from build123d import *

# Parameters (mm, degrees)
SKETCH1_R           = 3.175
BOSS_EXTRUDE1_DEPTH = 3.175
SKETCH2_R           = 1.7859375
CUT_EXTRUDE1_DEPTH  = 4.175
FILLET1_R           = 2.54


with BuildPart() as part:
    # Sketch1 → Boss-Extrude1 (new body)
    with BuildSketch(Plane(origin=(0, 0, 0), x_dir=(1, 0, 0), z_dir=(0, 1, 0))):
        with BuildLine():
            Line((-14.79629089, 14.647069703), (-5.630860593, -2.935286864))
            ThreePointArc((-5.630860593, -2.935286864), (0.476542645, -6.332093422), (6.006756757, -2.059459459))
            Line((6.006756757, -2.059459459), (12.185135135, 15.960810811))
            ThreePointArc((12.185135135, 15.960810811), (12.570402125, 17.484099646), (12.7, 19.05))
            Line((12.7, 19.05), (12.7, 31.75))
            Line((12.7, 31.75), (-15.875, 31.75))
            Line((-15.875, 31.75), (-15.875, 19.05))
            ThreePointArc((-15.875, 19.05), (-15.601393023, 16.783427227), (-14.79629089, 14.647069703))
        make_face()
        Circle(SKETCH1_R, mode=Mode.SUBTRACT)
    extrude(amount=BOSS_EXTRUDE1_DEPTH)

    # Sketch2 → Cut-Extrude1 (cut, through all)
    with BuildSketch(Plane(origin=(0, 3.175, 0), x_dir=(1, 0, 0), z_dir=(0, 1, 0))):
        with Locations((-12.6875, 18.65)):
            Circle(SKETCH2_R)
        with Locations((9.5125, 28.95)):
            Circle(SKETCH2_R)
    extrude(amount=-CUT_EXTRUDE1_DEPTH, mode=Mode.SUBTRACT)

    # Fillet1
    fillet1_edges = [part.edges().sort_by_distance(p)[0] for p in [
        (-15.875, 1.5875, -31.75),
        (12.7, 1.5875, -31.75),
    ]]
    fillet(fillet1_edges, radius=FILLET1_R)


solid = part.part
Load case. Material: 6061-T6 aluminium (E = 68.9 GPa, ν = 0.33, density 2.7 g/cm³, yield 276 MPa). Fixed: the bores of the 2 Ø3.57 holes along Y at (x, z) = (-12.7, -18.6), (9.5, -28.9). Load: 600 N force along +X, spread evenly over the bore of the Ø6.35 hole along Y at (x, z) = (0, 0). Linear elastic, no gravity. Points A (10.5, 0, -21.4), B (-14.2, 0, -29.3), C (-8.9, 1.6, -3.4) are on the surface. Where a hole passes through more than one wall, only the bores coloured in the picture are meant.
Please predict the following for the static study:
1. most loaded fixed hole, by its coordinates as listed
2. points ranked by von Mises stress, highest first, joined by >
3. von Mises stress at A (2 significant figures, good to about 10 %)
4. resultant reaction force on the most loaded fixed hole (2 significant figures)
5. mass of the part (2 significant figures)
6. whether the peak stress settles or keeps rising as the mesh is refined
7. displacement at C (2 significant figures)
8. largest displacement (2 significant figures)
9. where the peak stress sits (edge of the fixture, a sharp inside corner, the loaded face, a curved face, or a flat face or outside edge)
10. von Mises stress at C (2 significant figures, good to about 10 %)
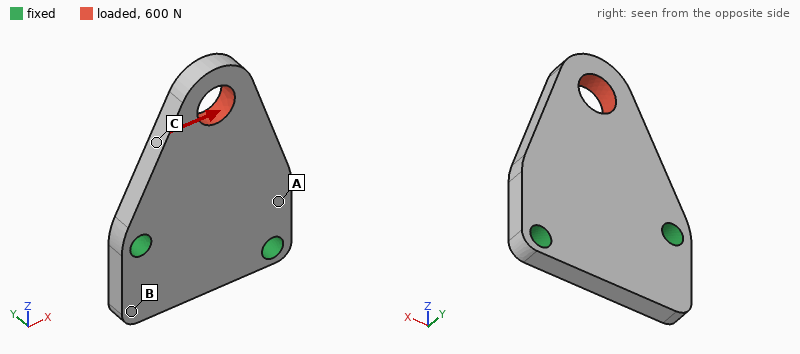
(-12.7, -18.6)
C > A > B
21 MPa
730 N
6.8 g
keeps rising
11 µm
22 µm
edge of the fixture
34 MPa
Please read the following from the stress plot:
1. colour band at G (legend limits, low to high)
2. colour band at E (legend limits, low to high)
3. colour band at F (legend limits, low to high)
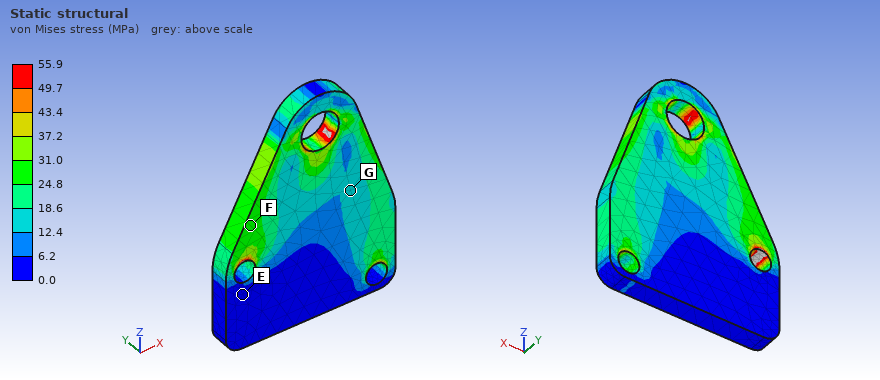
12.4 to 18.6 MPa
0.0 to 6.2 MPa
24.8 to 31.0 MPa
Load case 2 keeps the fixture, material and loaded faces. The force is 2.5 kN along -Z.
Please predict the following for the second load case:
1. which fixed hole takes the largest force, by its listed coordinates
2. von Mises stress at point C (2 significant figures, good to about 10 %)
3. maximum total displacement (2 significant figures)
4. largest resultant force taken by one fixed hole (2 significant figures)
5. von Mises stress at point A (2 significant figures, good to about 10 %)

(9.5, -28.9)
36 MPa
28 µm
1.5 kN
48 MPa
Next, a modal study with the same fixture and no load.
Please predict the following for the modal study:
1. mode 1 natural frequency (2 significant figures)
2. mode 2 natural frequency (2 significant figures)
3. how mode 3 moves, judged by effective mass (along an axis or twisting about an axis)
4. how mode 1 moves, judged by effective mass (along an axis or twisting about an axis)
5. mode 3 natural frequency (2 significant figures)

4500 Hz
13 kHz
along Y
along Y
19 kHz
